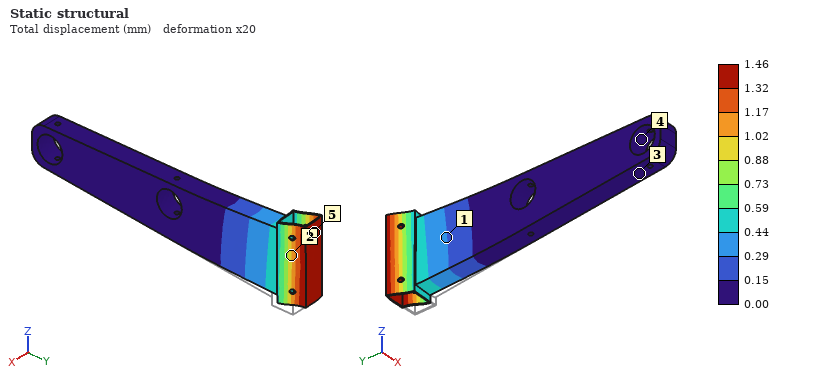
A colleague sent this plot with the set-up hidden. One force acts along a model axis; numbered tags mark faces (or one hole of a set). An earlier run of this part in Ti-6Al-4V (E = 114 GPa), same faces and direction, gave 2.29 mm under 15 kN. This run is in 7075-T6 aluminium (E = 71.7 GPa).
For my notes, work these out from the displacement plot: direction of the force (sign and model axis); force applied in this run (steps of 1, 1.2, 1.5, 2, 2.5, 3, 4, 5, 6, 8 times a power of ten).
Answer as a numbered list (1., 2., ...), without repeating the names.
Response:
1. -X
2. 6 kN
